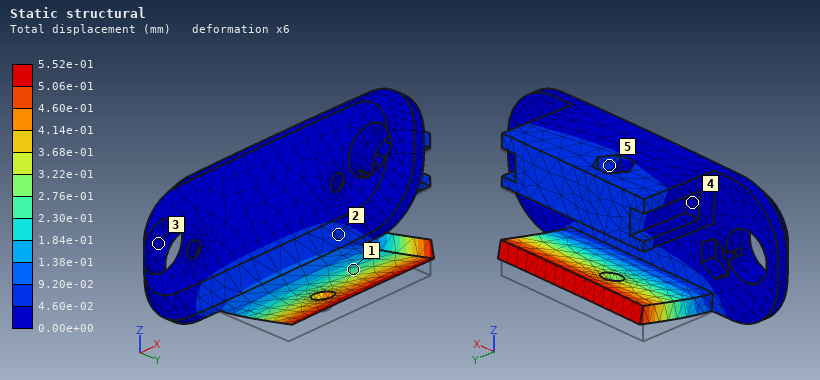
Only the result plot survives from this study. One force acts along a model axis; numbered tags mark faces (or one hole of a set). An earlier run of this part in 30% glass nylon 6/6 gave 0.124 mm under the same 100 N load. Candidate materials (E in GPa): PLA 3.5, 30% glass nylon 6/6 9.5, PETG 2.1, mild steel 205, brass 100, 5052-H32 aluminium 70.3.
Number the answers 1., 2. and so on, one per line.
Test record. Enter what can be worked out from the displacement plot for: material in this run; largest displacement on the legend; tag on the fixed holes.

1. PETG
2. 5.52e-01 mm
3. 3
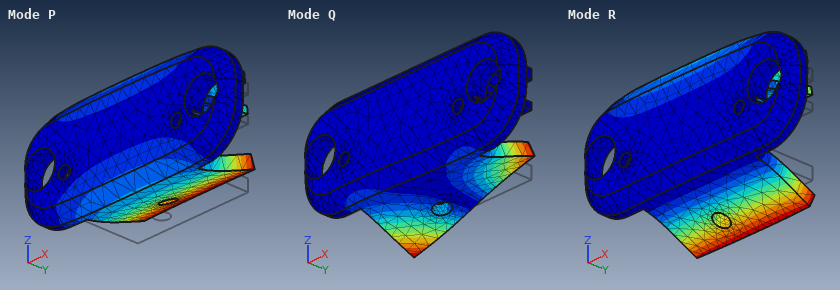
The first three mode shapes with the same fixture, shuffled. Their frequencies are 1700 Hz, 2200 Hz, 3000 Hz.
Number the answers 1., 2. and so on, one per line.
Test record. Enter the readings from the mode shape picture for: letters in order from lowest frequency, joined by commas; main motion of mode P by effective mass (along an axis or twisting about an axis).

1. P, R, Q
2. along Z
